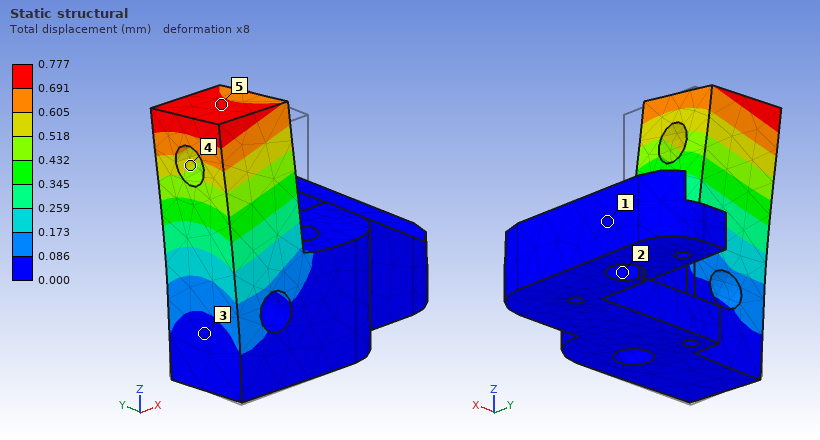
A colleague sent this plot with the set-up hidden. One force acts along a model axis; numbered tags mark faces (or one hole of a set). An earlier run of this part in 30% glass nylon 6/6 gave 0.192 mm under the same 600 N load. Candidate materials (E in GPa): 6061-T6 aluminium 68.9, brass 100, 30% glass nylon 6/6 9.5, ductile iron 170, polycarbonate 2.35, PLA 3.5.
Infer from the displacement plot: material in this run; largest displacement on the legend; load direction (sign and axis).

polycarbonate
0.777 mm
+Y
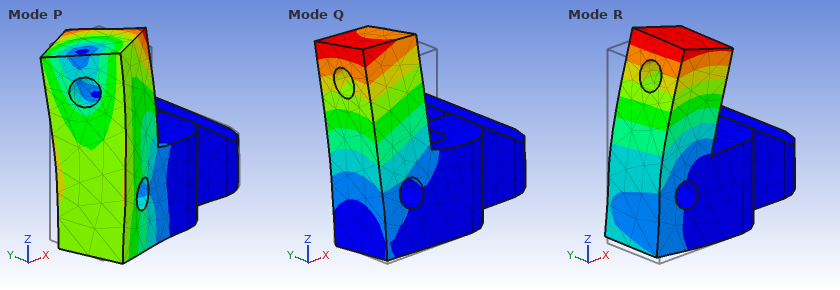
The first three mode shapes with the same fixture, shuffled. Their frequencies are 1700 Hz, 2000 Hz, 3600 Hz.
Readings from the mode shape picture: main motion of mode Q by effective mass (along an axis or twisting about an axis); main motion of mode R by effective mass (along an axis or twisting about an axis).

along Y
along X
